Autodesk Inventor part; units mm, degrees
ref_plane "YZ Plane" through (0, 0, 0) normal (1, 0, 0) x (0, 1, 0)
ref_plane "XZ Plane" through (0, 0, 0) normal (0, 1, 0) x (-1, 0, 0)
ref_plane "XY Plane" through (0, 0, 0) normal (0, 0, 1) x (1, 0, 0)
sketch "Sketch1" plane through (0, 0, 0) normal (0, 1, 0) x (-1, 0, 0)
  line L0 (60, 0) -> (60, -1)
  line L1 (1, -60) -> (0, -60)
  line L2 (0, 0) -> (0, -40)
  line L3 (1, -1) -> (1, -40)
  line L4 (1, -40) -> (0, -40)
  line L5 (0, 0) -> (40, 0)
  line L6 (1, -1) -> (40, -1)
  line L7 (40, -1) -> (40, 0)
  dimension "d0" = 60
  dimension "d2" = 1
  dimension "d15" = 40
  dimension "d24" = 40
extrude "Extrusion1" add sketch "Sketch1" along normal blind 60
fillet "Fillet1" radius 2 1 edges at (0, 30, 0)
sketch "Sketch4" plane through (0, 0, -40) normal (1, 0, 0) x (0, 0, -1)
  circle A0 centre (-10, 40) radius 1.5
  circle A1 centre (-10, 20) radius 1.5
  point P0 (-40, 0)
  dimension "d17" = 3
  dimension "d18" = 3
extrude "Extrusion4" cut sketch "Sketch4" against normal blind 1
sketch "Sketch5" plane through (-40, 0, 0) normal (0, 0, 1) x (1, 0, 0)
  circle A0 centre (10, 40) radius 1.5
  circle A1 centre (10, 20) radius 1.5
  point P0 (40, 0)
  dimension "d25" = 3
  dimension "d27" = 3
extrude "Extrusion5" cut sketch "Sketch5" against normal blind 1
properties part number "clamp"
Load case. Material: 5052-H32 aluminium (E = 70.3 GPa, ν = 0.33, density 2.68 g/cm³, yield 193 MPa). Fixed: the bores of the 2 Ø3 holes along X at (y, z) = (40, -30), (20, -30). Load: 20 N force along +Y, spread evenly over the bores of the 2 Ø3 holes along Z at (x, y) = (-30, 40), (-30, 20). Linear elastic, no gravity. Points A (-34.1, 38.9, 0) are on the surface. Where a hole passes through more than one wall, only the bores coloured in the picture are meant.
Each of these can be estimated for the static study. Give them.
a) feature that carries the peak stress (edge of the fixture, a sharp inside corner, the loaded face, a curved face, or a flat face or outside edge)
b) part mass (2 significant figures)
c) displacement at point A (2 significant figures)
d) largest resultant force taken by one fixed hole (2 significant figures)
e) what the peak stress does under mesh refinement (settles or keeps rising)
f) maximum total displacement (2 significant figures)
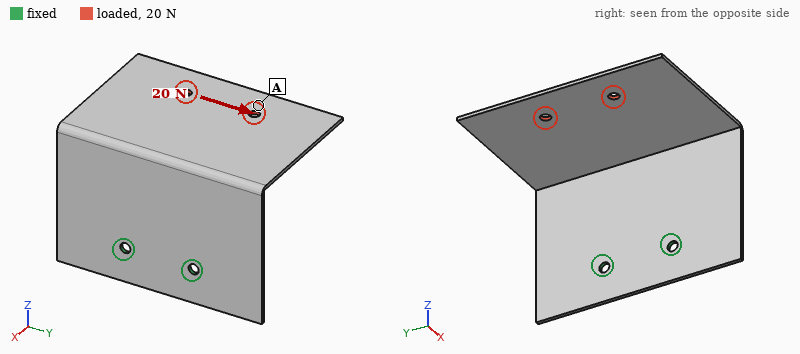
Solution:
edge of the fixture
12 g
0.68 mm
34 N
keeps rising
0.99 mm
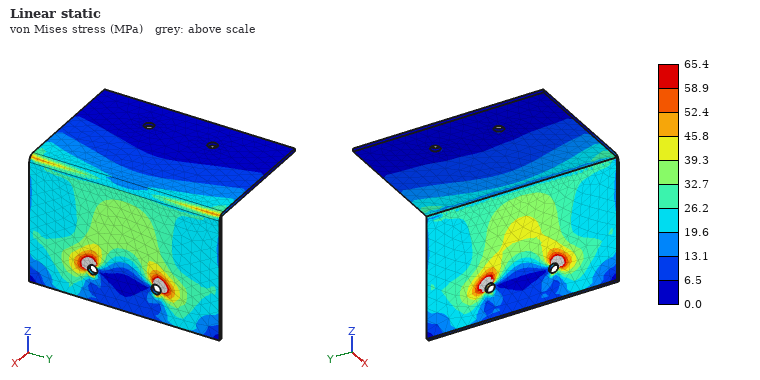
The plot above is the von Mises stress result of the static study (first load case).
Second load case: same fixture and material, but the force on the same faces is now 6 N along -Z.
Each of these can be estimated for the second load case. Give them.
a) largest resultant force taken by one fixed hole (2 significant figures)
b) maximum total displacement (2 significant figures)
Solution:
3.0 N
0.86 mm
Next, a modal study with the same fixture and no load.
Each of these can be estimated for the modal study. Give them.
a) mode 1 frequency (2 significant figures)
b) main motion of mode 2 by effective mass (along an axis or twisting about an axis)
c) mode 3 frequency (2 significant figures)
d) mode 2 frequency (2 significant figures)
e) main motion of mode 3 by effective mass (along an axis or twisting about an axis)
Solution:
230 Hz
along Y
610 Hz
360 Hz
along X
